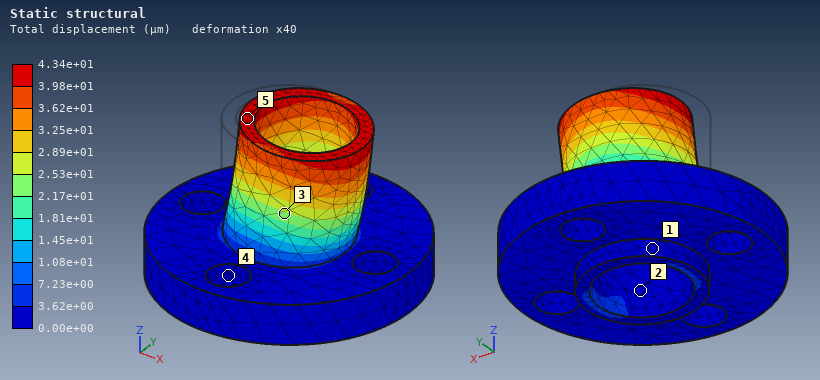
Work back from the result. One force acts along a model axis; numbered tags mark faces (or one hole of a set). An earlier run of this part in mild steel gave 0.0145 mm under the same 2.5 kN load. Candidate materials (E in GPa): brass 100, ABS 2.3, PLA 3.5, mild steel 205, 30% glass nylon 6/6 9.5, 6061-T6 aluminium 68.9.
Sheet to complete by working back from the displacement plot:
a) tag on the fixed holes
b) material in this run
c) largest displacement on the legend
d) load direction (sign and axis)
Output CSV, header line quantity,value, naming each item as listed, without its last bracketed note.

quantity,value
tag on the fixed holes,4
material in this run,6061-T6 aluminium
largest displacement on the legend,4.34e+01 µm
load direction,+X
